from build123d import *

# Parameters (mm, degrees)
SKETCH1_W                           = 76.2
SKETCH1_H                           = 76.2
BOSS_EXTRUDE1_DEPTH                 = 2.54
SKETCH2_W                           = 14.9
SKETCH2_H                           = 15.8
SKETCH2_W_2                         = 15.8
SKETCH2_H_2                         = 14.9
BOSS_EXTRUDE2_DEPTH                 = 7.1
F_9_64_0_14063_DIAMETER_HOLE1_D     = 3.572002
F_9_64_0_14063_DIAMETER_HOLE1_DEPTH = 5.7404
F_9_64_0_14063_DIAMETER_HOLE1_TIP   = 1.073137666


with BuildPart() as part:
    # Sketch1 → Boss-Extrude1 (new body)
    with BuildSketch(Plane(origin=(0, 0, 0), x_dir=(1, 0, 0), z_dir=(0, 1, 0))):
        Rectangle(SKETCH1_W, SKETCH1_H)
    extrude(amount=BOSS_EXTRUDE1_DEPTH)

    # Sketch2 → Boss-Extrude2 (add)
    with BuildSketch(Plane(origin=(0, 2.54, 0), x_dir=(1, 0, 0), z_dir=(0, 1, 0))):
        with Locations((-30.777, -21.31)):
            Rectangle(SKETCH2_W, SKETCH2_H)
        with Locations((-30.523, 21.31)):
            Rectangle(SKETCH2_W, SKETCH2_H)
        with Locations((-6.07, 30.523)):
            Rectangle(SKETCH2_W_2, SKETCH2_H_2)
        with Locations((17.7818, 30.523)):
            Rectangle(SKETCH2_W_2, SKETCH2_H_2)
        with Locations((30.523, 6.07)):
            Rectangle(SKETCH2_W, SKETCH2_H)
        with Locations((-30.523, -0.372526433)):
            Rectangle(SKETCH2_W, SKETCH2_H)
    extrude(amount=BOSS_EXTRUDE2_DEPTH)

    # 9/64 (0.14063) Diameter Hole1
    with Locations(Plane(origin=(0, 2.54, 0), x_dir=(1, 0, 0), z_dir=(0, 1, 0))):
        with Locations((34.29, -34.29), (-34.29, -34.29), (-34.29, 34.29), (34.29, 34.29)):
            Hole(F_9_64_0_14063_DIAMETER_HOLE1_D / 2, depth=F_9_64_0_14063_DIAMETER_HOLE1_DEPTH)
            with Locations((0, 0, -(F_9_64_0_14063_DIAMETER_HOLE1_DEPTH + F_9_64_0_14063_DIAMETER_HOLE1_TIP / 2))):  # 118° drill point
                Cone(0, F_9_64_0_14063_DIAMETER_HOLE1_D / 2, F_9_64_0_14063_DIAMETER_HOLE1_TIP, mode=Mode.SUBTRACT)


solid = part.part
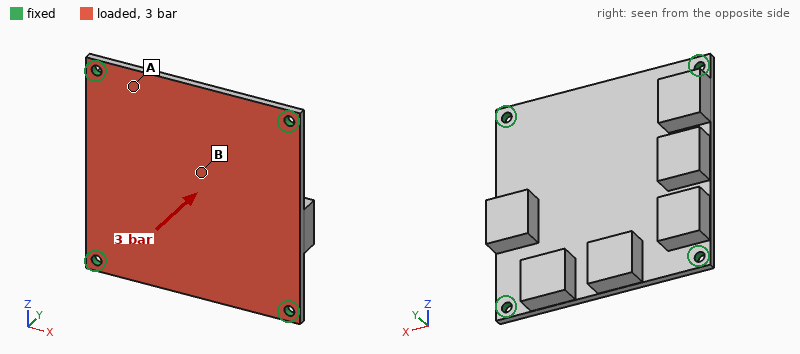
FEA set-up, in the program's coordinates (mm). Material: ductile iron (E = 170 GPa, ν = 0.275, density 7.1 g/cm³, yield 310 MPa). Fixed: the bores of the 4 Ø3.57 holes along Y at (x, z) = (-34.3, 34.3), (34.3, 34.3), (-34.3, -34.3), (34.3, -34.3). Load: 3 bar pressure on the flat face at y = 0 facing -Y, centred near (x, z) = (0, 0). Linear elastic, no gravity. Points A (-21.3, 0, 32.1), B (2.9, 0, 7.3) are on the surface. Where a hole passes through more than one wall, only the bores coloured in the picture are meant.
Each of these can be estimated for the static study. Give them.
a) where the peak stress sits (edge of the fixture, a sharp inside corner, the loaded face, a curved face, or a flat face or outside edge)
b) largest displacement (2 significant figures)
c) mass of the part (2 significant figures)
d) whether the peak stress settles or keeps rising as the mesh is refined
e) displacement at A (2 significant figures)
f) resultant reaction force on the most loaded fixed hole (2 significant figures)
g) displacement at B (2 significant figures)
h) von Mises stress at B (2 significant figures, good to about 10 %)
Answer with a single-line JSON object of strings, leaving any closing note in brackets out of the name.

{"where the peak stress sits": "edge of the fixture", "largest displacement": "0.17 mm", "mass of the part": "180 g", "whether the peak stress settles or keeps rising as the mesh is refined": "keeps rising", "displacement at A": "0.047 mm", "resultant reaction force on the most loaded fixed hole": "470 N", "displacement at B": "0.17 mm", "von Mises stress at B": "62 MPa"}
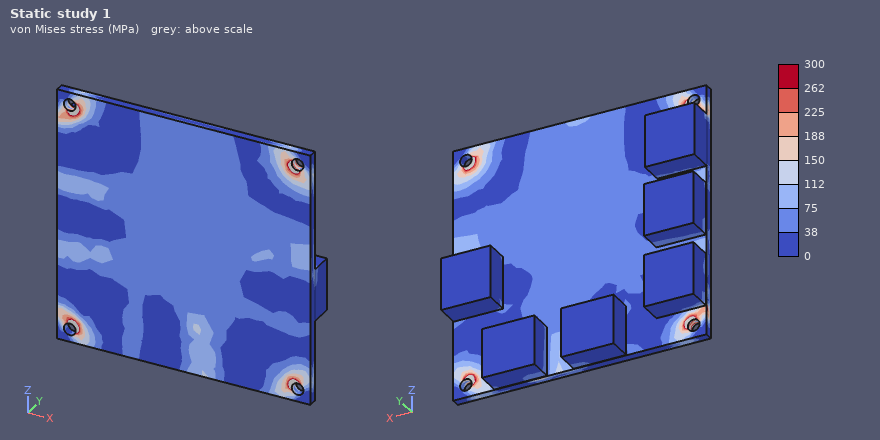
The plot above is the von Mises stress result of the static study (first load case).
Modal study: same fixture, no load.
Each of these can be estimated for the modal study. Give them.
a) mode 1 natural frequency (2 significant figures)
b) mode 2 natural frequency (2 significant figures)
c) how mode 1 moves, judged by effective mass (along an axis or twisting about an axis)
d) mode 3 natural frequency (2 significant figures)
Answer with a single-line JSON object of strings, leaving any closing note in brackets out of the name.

{"mode 1 natural frequency": "1600 Hz", "mode 2 natural frequency": "2600 Hz", "how mode 1 moves, judged by effective mass": "along Y", "mode 3 natural frequency": "2700 Hz"}
